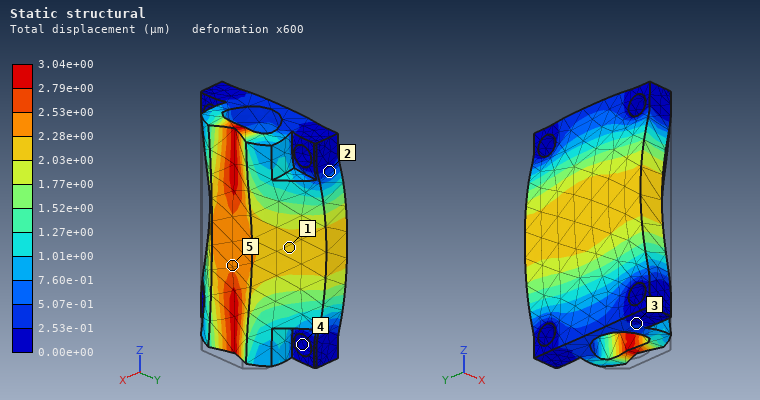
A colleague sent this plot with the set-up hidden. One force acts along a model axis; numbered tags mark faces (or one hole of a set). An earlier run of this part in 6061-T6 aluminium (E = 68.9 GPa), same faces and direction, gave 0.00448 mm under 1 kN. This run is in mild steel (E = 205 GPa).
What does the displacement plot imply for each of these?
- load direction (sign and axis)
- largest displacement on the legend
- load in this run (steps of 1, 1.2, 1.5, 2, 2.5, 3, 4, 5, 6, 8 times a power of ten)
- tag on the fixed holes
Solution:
-X
3.04e+00 µm
2 kN
4
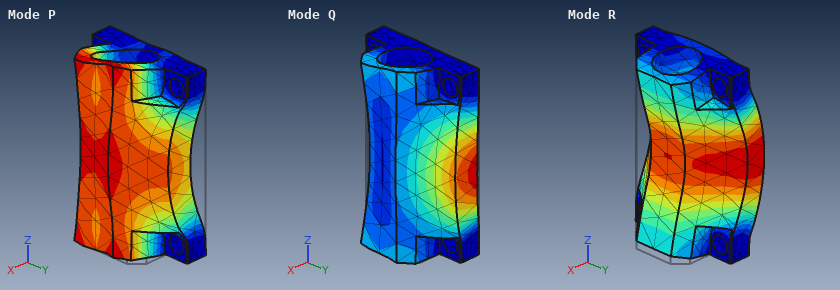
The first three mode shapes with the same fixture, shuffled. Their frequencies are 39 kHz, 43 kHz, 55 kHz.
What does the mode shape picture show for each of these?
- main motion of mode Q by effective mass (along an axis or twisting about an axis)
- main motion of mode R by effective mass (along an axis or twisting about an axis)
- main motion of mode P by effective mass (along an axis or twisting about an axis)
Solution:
along Y
along X
along Y
